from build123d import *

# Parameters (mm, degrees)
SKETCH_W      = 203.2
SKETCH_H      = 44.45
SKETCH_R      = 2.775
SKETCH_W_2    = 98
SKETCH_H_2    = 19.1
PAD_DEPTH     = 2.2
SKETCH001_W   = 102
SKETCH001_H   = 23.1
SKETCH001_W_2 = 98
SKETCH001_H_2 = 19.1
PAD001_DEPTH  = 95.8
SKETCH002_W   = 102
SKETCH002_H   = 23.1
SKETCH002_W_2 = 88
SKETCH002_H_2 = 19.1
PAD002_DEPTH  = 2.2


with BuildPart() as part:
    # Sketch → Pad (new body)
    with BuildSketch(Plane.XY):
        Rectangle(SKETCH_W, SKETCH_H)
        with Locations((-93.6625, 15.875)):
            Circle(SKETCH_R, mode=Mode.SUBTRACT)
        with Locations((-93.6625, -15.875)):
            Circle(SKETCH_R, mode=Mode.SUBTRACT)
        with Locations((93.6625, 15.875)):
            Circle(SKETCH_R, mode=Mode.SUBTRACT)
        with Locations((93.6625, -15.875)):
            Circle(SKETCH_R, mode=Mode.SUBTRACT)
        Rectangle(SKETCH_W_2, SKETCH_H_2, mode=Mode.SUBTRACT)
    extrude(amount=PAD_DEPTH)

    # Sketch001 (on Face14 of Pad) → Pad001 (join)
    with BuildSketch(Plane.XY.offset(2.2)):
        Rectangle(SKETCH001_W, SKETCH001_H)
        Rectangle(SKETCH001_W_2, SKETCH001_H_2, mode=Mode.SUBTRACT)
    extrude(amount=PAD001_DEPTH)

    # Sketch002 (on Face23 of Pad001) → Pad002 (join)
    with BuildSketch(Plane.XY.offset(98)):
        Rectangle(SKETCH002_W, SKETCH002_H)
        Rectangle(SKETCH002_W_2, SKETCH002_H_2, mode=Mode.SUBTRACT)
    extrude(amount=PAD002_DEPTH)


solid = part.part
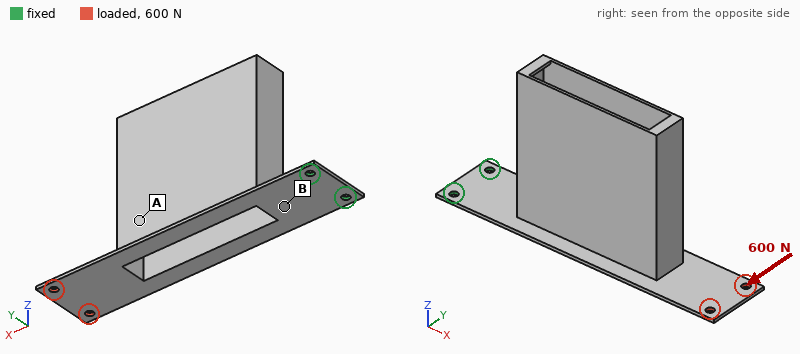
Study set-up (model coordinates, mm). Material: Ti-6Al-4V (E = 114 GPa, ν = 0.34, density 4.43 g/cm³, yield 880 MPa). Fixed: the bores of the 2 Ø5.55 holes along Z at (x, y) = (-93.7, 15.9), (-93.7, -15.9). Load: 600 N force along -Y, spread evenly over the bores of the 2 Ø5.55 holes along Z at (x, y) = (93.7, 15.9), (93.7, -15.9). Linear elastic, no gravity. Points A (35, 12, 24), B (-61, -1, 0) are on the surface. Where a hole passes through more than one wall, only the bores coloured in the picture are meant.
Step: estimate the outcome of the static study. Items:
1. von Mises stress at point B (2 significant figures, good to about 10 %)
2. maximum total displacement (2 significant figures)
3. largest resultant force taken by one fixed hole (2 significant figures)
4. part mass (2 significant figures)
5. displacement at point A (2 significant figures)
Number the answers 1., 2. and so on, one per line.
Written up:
1. 54 MPa
2. 1.2 mm
3. 3.4 kN
4. 280 g
5. 0.77 mm
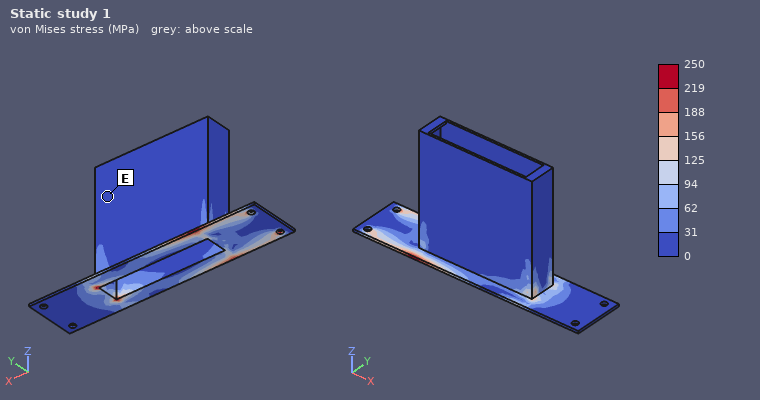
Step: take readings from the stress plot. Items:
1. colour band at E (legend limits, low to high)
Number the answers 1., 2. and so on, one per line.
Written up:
1. 0 to 31 MPa
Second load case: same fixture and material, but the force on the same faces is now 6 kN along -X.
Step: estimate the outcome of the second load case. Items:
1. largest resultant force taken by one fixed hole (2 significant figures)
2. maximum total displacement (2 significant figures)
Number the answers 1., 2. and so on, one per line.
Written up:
1. 3.0 kN
2. 0.53 mm
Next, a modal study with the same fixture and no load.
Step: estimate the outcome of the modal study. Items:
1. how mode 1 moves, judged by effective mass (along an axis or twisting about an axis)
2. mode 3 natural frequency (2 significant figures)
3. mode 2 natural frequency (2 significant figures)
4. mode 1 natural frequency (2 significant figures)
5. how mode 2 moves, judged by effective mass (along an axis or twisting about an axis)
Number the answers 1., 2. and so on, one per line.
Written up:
1. along Z
2. 380 Hz
3. 93 Hz
4. 32 Hz
5. along Y
